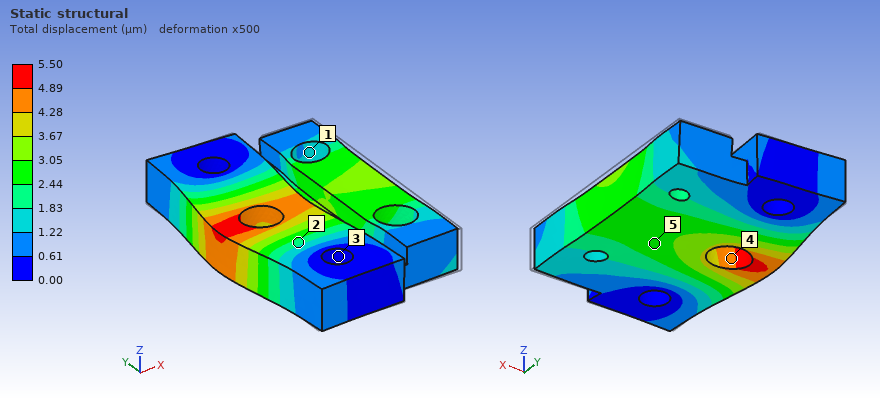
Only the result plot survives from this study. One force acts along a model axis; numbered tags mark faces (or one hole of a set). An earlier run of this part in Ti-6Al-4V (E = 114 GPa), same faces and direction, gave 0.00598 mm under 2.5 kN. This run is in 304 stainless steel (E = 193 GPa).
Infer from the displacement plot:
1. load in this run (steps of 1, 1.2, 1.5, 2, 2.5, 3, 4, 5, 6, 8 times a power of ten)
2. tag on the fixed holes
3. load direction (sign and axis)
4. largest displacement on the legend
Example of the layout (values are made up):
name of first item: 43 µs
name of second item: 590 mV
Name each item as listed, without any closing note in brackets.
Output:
load in this run: 4 kN
tag on the fixed holes: 3
load direction: -X
largest displacement on the legend: 5.50 µm
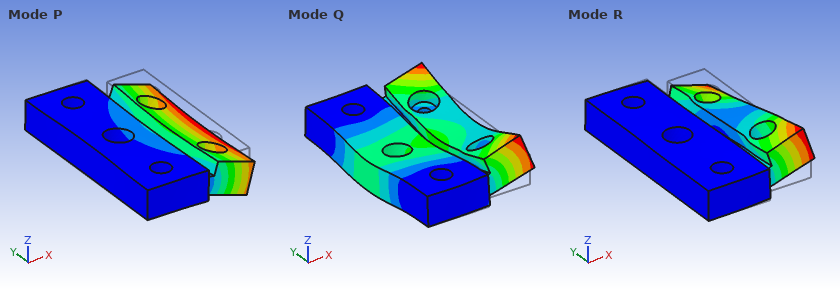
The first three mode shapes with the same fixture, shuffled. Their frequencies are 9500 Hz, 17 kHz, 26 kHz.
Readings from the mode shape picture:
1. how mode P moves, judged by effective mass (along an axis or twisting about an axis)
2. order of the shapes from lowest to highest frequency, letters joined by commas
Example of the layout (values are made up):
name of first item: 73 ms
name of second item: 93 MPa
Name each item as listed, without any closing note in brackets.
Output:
how mode P moves, judged by effective mass: along Z
order of the shapes from lowest to highest frequency, letters joined by commas: P, R, Q
